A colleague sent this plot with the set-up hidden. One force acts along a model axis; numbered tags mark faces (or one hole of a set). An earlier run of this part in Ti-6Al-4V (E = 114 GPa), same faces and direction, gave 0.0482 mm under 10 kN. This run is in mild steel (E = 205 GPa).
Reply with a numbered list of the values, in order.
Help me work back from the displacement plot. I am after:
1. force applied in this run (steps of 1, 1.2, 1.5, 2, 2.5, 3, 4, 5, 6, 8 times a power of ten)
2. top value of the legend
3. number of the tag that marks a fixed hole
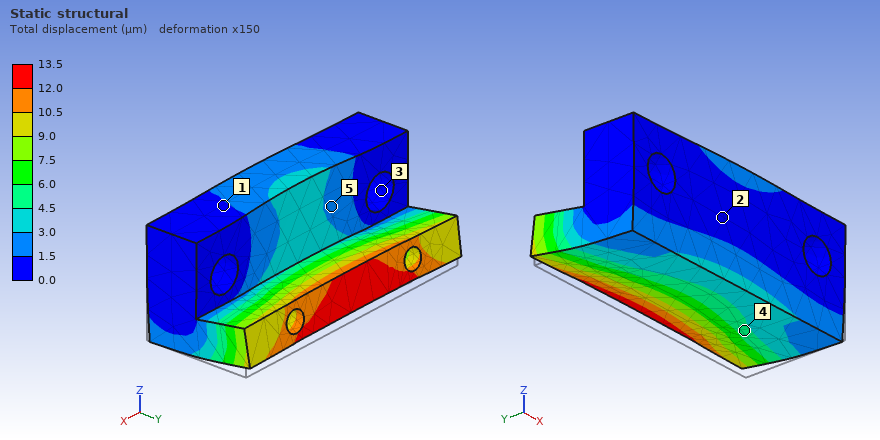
1. 5 kN
2. 13.5 µm
3. 3
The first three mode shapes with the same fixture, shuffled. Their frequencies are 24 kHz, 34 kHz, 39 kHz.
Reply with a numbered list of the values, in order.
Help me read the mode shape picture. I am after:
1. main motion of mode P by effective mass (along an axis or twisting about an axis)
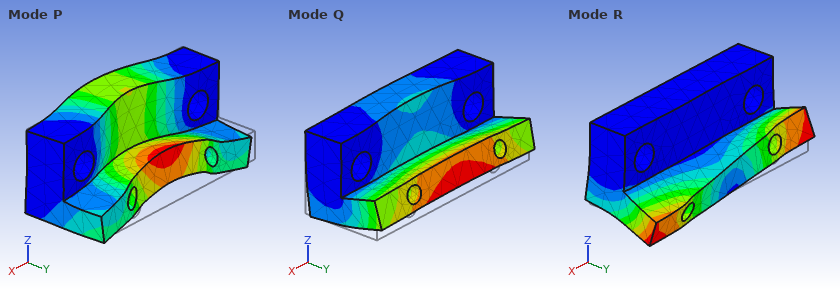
1. along Y
